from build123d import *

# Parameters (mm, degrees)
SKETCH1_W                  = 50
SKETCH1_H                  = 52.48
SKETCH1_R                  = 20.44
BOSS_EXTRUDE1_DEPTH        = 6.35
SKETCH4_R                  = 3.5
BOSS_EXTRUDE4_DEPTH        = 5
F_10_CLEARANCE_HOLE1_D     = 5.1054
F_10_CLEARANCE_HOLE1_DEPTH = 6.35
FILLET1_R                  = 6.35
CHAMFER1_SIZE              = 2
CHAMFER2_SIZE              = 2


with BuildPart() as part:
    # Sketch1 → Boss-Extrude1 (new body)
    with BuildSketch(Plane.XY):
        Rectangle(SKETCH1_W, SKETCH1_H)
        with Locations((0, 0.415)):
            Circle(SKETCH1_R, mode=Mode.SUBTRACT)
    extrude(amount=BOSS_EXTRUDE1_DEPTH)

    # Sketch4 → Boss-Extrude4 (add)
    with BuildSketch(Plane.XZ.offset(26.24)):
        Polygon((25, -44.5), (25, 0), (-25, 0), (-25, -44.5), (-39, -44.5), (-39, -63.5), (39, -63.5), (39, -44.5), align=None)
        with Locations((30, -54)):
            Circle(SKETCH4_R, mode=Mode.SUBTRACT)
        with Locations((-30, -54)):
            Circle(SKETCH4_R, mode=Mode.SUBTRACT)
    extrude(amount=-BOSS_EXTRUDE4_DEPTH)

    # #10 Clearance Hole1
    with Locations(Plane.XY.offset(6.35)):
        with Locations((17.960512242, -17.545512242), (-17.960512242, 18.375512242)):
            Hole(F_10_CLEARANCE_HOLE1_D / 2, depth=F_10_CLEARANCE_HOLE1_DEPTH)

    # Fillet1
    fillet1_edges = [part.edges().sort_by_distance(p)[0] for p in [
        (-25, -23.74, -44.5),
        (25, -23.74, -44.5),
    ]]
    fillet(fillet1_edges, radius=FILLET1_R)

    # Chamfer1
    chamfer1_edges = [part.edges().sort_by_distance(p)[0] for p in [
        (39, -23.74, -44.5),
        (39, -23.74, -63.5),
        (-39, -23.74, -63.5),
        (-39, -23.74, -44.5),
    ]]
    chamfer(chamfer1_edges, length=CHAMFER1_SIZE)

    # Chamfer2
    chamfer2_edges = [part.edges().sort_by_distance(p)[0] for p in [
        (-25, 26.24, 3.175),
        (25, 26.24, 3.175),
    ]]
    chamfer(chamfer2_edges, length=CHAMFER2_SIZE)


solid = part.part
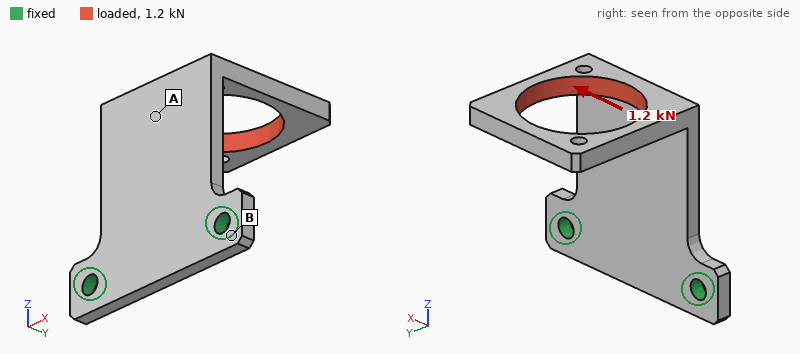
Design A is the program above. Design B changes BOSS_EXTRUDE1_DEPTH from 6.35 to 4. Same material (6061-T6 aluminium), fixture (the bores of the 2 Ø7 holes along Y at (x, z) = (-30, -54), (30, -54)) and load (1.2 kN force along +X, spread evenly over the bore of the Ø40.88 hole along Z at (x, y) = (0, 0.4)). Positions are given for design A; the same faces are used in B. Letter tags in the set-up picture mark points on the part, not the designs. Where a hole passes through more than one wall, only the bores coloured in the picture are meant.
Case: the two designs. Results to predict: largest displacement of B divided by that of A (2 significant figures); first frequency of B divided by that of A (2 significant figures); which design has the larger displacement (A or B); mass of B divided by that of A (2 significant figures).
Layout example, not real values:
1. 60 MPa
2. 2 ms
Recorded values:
1. 1.1
2. 1.1
3. B
4. 0.89
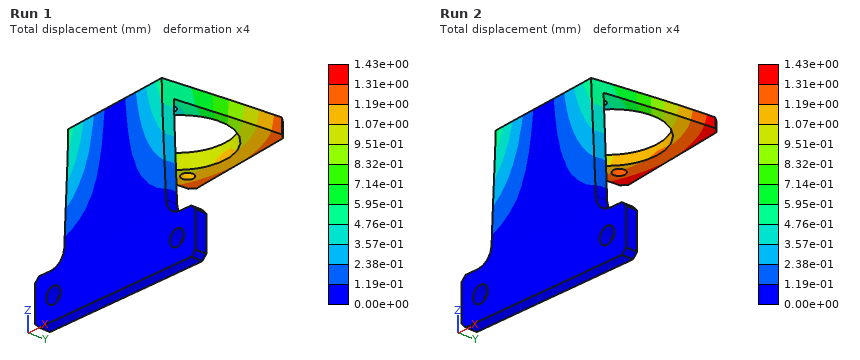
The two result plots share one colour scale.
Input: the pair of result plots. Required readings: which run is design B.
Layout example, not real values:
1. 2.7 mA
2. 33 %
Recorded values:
1. Run 2
